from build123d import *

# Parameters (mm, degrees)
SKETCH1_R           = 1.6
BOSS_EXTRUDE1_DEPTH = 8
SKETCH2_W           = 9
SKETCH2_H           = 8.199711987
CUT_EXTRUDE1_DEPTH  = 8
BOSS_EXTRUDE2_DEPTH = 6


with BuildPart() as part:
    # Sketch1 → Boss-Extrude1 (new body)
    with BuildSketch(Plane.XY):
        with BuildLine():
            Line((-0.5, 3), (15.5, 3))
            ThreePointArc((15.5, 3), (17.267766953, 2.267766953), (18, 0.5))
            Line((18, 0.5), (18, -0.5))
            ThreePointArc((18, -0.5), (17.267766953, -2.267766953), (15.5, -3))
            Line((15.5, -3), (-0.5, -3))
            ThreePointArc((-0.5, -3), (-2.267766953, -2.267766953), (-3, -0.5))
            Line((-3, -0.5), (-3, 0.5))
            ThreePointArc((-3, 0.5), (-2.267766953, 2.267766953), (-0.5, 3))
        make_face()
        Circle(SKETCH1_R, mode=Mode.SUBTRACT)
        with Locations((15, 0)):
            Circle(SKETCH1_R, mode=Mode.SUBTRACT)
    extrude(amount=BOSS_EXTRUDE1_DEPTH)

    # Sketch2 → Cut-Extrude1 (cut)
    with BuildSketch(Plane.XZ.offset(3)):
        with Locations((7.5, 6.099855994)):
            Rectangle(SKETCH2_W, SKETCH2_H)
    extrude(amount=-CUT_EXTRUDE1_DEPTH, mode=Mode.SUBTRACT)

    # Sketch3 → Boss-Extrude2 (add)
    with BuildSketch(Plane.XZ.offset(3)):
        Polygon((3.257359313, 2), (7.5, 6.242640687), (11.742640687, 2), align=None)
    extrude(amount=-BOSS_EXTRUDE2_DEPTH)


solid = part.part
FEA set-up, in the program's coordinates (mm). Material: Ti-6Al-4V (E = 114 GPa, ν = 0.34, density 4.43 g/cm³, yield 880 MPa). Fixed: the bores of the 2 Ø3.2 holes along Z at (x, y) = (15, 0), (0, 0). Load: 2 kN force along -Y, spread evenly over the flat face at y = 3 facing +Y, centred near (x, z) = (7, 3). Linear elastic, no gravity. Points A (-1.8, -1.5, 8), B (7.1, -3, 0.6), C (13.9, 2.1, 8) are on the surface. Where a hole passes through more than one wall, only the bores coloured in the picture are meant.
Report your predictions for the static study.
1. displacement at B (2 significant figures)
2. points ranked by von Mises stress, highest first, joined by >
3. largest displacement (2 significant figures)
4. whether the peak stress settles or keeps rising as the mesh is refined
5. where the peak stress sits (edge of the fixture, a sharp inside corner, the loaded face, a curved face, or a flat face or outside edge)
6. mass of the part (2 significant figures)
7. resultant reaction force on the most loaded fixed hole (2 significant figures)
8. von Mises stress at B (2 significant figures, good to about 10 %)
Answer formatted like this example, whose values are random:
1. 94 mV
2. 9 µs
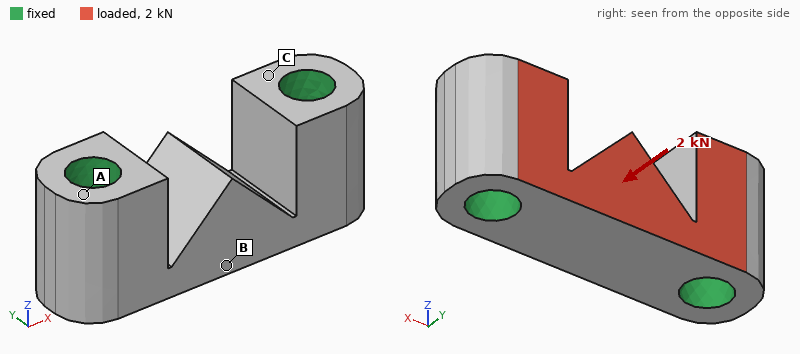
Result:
1. 4.7 µm
2. B > C > A
3. 11 µm
4. keeps rising
5. a sharp inside corner
6. 2.7 g
7. 1.0 kN
8. 57 MPa
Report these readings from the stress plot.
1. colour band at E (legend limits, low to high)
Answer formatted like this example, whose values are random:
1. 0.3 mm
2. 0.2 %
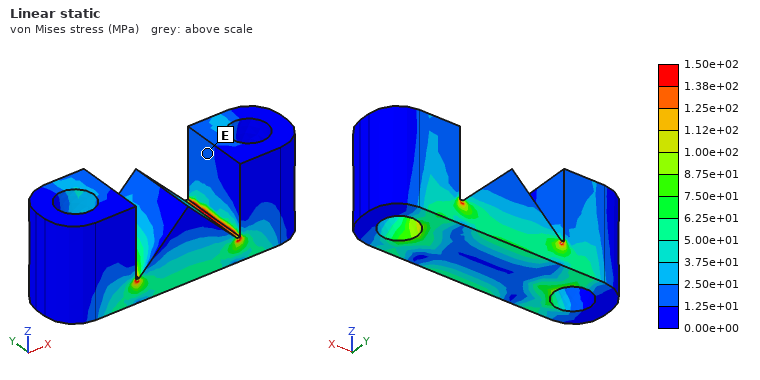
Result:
1. 1.25e+01 to 2.50e+01 MPa
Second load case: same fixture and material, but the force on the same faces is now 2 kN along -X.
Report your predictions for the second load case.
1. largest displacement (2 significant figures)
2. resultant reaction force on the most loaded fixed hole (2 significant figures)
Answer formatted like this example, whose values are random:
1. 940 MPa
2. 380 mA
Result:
1. 4.3 µm
2. 1.0 kN
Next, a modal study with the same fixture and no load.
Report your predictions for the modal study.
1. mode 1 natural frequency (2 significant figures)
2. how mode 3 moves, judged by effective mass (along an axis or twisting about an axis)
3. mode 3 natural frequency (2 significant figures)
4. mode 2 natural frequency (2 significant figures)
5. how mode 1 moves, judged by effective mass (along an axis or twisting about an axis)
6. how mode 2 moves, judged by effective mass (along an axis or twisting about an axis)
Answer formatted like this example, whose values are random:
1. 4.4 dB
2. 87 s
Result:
1. 54 kHz
2. along Y
3. 93 kHz
4. 73 kHz
5. along Y
6. along Z
